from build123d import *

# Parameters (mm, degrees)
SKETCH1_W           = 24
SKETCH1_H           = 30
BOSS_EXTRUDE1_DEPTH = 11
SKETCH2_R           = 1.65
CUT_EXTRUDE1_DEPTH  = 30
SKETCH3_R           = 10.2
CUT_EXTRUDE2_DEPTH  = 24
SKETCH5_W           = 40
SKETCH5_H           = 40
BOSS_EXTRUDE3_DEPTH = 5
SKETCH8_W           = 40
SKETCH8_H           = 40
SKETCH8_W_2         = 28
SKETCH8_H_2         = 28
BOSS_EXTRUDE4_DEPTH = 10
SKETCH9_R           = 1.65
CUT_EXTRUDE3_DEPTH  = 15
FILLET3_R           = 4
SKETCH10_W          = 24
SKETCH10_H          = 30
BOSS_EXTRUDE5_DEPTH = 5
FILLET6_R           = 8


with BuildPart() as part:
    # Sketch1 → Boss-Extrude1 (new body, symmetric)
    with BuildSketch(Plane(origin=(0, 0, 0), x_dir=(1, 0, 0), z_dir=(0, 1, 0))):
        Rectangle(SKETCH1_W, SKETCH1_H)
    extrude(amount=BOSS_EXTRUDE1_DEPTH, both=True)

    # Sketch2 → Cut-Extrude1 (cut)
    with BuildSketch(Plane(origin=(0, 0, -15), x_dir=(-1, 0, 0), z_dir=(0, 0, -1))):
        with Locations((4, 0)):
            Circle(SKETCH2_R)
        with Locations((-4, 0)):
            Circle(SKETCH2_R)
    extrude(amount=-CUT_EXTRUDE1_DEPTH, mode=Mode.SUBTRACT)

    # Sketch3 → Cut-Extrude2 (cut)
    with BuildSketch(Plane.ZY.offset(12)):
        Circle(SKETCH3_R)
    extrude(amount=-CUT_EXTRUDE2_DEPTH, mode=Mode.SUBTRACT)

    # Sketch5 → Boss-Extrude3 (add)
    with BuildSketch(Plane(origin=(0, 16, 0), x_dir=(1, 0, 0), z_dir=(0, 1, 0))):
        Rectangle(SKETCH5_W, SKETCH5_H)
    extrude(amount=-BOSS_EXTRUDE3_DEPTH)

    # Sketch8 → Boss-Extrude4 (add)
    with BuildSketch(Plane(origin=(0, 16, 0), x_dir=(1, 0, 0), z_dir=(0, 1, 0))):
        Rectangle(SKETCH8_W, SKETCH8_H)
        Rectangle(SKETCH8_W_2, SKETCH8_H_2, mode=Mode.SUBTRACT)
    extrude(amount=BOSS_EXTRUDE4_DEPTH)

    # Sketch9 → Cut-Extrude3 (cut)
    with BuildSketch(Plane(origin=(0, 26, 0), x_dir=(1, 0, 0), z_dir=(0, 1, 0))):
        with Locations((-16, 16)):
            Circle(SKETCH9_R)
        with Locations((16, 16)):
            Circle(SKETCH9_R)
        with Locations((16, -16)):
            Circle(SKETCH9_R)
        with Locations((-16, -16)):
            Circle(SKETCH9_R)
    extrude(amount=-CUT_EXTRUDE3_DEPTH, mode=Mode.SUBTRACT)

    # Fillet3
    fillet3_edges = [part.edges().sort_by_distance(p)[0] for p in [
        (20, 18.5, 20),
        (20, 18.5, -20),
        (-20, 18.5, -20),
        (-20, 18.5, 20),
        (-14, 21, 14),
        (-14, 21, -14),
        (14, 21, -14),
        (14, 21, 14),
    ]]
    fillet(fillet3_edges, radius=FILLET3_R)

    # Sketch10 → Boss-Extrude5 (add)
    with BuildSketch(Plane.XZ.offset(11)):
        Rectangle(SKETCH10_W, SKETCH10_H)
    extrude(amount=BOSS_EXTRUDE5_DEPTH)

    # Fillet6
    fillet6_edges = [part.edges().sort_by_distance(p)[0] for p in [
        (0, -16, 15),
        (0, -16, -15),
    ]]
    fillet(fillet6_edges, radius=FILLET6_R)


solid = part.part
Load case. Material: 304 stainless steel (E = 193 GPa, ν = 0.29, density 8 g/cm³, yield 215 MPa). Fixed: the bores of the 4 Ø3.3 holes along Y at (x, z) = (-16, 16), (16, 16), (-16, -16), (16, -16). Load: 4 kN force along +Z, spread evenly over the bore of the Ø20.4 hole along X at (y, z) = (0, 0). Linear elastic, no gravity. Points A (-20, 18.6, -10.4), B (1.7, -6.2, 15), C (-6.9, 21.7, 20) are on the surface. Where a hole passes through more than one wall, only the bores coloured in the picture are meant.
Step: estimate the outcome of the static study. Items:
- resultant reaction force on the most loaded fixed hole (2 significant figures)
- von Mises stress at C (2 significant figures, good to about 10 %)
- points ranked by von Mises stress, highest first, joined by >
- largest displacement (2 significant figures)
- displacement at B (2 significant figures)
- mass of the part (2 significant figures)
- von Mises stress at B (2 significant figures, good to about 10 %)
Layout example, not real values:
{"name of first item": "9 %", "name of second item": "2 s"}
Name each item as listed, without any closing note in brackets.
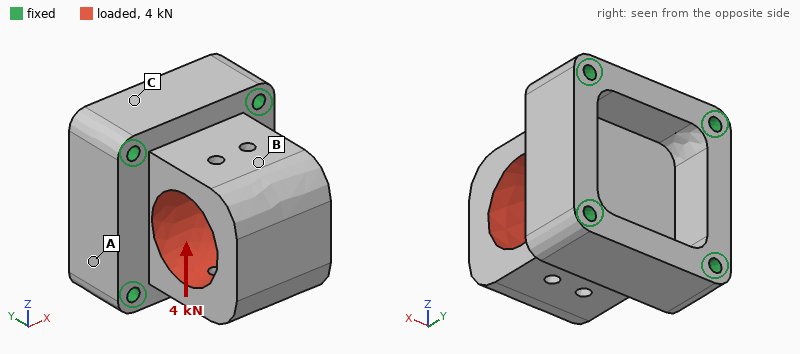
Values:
{"resultant reaction force on the most loaded fixed hole": "1.5 kN", "von Mises stress at C": "9.8 MPa", "points ranked by von Mises stress, highest first, joined by >": "B > C > A", "largest displacement": "14 µm", "displacement at B": "12 µm", "mass of the part": "210 g", "von Mises stress at B": "21 MPa"}
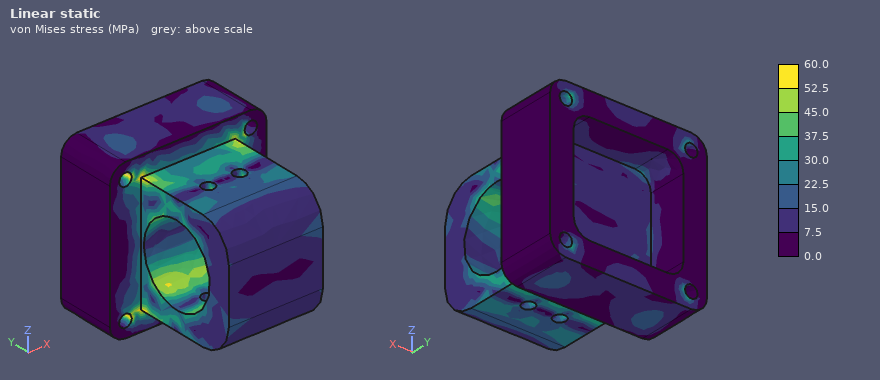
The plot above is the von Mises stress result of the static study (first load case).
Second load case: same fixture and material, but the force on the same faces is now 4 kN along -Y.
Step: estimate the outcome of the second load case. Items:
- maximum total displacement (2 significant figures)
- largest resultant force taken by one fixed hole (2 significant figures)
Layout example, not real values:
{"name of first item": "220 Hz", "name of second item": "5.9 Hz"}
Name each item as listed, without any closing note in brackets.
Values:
{"maximum total displacement": "3.3 µm", "largest resultant force taken by one fixed hole": "1.1 kN"}
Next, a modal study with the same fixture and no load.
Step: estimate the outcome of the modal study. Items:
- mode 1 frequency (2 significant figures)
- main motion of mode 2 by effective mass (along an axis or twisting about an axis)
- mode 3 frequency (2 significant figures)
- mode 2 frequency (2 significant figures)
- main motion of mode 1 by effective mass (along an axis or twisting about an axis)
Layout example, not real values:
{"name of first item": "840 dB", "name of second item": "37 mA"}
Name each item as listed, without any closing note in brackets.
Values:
{"mode 1 frequency": "8800 Hz", "main motion of mode 2 by effective mass": "along X", "mode 3 frequency": "16 kHz", "mode 2 frequency": "10 kHz", "main motion of mode 1 by effective mass": "along Z"}
